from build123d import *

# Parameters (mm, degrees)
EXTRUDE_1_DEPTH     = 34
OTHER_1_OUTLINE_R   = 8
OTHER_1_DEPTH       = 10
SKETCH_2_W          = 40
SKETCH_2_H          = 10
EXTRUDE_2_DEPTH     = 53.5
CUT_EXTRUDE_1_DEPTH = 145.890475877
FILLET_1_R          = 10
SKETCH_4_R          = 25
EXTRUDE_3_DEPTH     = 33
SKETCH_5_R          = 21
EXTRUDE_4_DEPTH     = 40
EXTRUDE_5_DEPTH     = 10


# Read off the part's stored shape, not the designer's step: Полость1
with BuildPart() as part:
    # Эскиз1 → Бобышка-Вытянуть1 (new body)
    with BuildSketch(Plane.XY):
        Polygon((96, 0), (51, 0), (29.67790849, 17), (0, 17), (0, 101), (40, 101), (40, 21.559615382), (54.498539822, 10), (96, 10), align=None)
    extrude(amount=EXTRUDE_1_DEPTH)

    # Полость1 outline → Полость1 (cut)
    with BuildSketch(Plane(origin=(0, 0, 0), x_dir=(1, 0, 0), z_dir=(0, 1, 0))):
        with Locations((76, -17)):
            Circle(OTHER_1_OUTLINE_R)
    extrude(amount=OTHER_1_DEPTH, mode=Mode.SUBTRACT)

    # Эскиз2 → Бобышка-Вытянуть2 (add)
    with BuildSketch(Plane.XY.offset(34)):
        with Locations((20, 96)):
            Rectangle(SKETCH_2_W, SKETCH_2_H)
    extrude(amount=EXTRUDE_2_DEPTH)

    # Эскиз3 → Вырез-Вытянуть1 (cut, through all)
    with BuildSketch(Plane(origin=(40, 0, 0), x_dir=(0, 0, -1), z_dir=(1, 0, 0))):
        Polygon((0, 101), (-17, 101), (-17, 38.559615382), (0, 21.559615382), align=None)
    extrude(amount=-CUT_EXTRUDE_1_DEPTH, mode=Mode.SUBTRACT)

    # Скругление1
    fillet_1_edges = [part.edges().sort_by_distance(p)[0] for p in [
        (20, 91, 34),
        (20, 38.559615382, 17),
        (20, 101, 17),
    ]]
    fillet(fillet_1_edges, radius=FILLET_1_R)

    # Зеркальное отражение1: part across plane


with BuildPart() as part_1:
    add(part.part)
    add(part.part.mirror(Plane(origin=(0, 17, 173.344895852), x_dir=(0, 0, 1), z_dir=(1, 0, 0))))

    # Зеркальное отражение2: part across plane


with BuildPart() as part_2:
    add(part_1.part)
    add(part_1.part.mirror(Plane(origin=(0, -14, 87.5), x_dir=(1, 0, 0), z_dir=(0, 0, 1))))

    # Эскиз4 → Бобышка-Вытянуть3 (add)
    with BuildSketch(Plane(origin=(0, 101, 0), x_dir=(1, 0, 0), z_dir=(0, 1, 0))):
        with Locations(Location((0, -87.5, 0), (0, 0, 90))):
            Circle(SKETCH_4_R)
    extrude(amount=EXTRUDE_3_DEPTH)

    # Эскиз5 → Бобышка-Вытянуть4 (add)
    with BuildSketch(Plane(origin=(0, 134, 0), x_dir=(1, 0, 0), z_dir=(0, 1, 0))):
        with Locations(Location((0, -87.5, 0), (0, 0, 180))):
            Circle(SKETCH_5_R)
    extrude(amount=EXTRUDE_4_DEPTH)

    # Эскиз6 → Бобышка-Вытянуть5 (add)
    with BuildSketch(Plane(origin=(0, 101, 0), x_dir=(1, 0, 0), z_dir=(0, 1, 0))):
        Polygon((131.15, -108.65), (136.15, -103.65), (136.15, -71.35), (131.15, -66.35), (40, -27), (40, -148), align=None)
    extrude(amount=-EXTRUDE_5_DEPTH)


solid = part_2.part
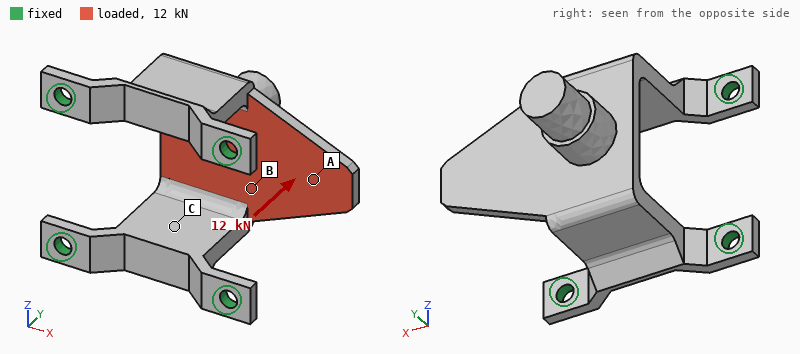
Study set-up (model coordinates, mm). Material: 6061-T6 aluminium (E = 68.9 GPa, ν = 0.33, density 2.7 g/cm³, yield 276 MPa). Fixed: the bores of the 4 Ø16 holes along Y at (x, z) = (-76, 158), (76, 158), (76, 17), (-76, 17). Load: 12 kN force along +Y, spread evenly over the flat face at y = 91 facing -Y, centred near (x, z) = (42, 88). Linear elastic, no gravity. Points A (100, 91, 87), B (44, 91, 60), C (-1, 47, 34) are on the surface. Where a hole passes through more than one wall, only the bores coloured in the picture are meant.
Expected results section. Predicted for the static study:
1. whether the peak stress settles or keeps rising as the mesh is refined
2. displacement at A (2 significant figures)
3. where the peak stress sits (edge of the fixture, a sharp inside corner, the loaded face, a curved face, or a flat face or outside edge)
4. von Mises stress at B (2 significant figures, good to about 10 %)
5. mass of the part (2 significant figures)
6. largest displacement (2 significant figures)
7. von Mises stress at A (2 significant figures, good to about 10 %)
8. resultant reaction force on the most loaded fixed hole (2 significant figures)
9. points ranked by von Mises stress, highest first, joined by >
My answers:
keeps rising
1.3 mm
a sharp inside corner
110 MPa
1.7 kg
2.1 mm
43 MPa
6.8 kN
B > A > C
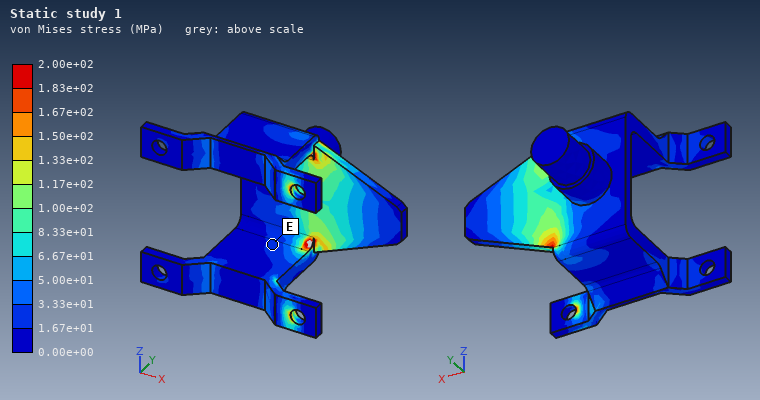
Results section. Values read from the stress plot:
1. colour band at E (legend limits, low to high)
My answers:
1.67e+01 to 3.33e+01 MPa
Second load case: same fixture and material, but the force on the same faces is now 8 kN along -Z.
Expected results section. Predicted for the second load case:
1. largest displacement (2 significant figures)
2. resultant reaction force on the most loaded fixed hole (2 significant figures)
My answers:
0.66 mm
4.5 kN
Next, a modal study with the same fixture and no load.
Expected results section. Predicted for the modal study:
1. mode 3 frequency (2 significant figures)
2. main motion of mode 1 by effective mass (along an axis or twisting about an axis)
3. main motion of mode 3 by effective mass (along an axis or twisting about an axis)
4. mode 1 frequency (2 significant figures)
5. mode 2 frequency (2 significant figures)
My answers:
1100 Hz
along Z
along X
640 Hz
720 Hz
